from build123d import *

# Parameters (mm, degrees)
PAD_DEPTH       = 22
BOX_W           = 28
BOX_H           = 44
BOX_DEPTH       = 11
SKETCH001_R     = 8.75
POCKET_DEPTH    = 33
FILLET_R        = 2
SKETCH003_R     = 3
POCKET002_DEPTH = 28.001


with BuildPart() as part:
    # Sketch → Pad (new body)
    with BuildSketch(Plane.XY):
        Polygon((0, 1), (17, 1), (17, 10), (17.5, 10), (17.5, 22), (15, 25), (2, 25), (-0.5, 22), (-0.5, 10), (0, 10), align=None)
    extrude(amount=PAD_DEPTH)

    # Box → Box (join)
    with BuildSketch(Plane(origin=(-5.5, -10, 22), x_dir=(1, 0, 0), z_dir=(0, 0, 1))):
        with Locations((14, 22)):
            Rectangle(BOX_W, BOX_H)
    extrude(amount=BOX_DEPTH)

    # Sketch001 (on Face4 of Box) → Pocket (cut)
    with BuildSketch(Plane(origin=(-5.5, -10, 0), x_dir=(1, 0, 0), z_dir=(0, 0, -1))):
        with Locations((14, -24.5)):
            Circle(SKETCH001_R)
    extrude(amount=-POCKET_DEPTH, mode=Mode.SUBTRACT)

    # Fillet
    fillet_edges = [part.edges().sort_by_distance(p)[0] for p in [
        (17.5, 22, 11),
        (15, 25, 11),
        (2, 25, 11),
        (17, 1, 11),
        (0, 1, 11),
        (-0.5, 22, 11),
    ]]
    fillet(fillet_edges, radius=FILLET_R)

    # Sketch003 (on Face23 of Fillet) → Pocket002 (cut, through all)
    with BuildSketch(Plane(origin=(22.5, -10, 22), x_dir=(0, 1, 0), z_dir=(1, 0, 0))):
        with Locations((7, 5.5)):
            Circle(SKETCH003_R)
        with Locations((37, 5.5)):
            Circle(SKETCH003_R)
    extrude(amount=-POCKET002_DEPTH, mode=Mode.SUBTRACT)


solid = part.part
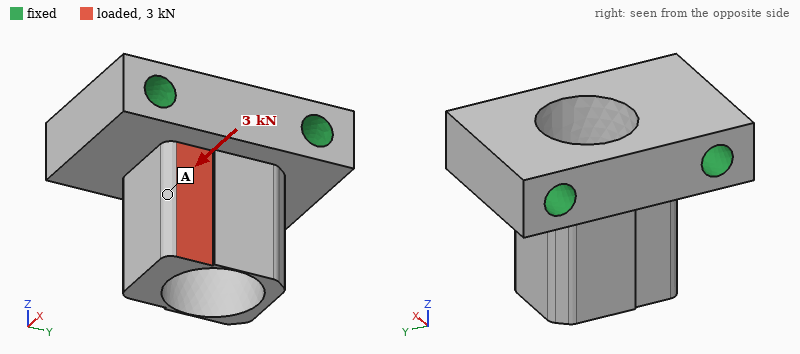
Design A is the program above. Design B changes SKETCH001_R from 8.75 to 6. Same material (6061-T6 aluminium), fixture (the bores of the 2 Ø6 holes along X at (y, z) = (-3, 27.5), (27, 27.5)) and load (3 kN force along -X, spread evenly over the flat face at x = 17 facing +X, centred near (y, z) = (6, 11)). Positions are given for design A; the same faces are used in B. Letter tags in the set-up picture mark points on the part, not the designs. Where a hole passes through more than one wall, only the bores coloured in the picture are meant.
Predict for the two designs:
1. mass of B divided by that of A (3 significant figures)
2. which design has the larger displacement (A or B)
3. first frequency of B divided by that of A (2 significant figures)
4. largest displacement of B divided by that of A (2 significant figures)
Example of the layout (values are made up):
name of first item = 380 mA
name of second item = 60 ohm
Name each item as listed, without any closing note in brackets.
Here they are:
mass of B divided by that of A = 1.32
which design has the larger displacement = A
first frequency of B divided by that of A = 0.97
largest displacement of B divided by that of A = 0.36
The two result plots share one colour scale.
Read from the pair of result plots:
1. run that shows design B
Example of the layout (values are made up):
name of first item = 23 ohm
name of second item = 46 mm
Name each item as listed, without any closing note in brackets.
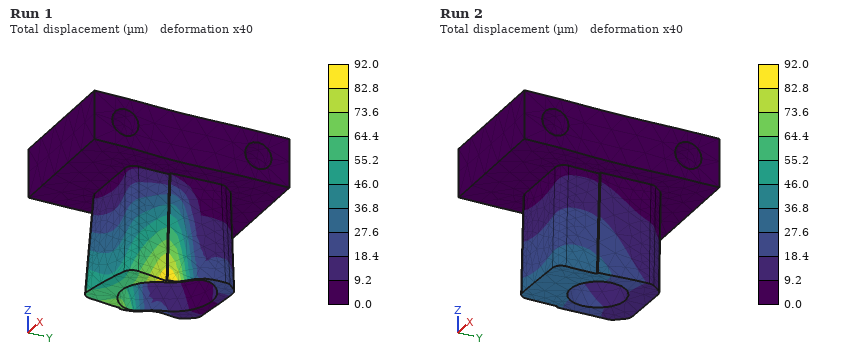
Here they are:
run that shows design B = Run 2
